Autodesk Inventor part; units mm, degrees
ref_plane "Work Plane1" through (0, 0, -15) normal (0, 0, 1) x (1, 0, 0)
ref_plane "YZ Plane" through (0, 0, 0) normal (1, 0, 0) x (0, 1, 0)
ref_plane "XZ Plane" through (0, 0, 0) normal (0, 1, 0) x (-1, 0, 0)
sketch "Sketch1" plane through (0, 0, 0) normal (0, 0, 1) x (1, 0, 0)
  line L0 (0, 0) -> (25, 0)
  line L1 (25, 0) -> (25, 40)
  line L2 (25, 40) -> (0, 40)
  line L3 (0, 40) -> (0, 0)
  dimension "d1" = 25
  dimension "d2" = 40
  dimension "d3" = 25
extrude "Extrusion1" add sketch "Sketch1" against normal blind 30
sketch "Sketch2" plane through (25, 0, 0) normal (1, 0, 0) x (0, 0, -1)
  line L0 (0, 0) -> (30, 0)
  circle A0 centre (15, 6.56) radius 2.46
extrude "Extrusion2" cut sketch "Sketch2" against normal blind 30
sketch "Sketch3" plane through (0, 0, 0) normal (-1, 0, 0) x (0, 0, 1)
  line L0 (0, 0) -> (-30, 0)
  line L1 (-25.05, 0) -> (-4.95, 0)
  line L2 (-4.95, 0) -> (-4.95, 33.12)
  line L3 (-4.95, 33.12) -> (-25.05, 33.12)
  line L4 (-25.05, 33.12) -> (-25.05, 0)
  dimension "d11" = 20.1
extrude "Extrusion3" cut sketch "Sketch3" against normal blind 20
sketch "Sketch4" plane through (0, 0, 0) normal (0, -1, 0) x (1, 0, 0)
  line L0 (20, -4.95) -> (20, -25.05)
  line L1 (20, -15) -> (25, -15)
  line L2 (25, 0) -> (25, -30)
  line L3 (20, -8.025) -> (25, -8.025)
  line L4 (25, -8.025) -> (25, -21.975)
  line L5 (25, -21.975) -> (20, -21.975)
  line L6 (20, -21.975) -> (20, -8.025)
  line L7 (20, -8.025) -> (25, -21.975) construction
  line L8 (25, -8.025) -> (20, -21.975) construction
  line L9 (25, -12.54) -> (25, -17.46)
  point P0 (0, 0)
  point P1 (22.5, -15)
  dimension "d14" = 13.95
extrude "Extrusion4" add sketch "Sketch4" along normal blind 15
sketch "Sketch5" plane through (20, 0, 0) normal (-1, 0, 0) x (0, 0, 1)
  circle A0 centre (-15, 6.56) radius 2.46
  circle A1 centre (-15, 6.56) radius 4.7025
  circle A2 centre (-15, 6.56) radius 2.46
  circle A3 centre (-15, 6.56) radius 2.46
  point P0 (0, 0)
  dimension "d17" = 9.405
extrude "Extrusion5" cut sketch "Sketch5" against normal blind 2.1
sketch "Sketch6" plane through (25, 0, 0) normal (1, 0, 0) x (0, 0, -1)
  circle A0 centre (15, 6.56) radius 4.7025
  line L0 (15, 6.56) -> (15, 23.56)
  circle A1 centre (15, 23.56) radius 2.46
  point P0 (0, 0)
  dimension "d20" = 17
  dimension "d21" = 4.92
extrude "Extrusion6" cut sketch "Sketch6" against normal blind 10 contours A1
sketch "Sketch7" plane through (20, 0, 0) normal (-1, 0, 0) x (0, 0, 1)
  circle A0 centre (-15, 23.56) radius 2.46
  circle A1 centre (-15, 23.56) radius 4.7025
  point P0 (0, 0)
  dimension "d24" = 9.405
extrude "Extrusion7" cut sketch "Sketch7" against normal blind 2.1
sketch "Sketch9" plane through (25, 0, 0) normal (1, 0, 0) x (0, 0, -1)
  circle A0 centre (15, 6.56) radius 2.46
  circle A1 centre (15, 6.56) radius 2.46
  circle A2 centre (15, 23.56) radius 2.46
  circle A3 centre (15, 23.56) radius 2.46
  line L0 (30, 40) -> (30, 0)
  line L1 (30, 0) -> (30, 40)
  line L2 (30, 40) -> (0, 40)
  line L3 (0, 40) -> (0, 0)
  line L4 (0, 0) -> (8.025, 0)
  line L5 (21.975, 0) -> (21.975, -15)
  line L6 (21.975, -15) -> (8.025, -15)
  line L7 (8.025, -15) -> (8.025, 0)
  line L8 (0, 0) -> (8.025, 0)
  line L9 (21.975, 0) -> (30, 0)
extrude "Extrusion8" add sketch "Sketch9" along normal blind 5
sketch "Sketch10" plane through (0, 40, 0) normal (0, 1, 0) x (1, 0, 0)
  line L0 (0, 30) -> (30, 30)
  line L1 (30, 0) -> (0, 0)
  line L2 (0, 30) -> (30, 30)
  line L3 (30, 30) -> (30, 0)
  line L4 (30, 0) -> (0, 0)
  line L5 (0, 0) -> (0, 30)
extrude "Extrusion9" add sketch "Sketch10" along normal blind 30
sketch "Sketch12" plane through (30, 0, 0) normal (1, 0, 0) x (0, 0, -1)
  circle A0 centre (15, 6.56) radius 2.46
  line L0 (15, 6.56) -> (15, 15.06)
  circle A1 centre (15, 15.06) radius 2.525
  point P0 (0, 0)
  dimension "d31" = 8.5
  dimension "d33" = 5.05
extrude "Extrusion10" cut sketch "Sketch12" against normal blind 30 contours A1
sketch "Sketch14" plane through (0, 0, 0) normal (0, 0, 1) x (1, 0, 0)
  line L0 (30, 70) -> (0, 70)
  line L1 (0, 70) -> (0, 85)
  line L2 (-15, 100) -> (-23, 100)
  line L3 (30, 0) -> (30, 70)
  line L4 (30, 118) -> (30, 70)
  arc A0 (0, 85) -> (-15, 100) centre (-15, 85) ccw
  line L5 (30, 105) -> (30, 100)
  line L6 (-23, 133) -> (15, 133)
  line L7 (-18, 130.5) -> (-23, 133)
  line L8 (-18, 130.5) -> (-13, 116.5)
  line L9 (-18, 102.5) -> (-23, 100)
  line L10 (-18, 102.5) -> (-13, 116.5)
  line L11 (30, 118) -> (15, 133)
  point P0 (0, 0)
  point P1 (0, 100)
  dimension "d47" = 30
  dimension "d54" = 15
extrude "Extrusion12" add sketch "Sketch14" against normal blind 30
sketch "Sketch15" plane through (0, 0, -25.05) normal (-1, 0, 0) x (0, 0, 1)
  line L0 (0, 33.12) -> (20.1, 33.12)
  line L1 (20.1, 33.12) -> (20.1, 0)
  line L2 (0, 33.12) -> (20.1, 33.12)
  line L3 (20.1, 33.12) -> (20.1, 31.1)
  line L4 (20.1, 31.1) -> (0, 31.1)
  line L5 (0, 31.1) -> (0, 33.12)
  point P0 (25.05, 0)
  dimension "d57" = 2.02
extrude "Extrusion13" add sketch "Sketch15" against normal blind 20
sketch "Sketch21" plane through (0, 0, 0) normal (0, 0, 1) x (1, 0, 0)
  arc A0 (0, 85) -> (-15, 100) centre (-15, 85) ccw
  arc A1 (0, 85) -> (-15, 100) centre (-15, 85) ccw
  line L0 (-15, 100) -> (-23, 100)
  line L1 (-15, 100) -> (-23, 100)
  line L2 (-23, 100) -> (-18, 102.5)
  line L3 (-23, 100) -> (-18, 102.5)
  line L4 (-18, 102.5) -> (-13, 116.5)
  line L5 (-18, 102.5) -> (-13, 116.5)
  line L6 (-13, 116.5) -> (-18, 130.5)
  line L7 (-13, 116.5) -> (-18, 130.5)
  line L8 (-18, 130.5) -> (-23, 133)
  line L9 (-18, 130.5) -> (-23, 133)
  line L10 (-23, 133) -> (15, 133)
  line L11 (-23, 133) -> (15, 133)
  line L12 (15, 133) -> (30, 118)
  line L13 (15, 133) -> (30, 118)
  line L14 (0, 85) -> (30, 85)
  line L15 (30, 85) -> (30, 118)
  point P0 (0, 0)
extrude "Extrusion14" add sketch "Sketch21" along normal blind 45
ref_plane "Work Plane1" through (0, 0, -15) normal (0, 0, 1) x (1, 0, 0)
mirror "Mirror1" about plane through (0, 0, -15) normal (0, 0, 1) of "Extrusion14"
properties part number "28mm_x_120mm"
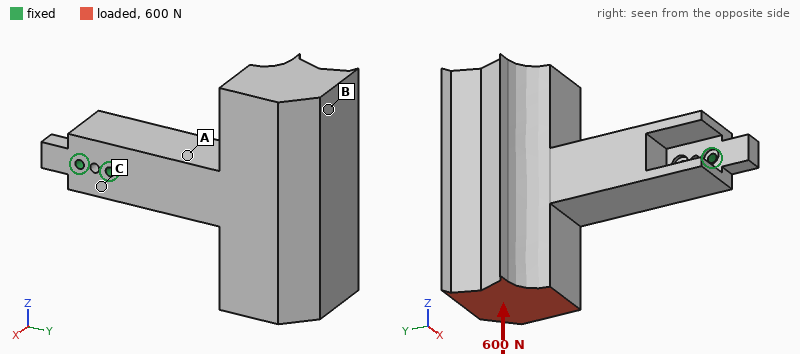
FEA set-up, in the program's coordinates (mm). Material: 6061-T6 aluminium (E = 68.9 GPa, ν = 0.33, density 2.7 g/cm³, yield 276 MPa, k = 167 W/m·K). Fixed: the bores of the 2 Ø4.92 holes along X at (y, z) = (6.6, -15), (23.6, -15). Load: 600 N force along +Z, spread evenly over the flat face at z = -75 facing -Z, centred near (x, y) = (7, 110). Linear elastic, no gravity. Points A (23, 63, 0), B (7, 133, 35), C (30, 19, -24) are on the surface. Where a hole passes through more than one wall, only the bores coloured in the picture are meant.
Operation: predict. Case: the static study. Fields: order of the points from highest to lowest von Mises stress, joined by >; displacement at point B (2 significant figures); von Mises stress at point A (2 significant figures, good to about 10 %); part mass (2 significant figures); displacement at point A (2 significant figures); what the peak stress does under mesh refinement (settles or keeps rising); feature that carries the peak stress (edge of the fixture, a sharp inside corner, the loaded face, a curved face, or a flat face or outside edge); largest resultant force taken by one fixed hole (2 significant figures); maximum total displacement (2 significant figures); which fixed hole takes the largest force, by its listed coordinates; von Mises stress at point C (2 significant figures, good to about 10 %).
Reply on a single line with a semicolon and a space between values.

C > A > B; 0.13 mm; 6.5 MPa; 800 g; 0.039 mm; keeps rising; edge of the fixture; 2.8 kN; 0.15 mm; (23.6, -15); 18 MPa
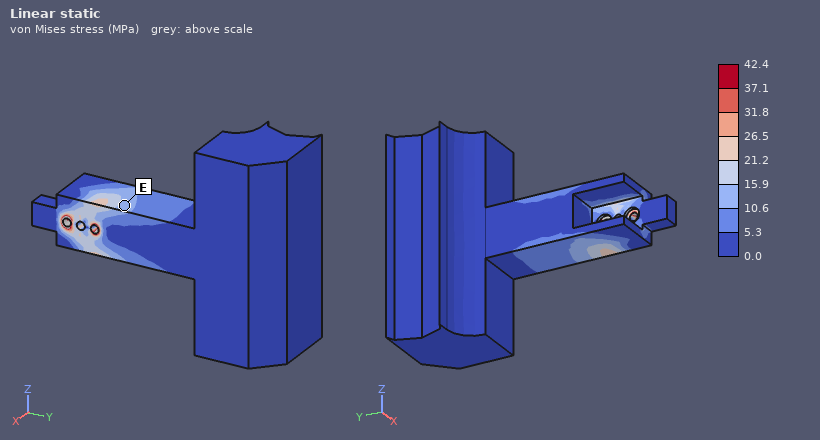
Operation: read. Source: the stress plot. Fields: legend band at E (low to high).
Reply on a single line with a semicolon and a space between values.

10.6 to 15.9 MPa
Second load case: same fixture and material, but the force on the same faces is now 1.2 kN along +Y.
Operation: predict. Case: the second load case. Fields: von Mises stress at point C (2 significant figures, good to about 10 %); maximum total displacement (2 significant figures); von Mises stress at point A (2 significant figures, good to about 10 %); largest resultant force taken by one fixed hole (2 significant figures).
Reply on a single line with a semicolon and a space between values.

18 MPa; 0.25 mm; 16 MPa; 3.3 kN
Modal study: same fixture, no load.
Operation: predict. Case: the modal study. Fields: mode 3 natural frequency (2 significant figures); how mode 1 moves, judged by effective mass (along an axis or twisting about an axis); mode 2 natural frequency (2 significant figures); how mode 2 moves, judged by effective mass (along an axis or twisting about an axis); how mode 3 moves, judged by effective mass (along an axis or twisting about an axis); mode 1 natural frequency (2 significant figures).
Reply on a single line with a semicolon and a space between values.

670 Hz; along X; 450 Hz; along Z; twisting about Y; 420 Hz
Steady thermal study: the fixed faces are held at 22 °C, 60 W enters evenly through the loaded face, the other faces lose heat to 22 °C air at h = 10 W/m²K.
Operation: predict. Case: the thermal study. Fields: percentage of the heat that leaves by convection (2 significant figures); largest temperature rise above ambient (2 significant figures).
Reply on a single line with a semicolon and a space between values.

17 %; 43 K
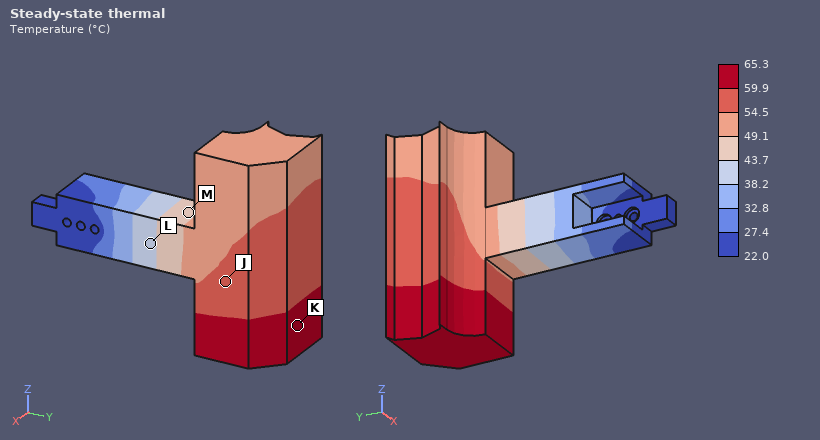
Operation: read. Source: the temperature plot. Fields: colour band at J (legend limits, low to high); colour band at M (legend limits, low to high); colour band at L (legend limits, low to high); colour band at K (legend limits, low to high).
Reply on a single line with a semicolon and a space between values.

54.5 to 59.9 °C; 43.7 to 49.1 °C; 38.2 to 43.7 °C; 59.9 to 65.3 °C
